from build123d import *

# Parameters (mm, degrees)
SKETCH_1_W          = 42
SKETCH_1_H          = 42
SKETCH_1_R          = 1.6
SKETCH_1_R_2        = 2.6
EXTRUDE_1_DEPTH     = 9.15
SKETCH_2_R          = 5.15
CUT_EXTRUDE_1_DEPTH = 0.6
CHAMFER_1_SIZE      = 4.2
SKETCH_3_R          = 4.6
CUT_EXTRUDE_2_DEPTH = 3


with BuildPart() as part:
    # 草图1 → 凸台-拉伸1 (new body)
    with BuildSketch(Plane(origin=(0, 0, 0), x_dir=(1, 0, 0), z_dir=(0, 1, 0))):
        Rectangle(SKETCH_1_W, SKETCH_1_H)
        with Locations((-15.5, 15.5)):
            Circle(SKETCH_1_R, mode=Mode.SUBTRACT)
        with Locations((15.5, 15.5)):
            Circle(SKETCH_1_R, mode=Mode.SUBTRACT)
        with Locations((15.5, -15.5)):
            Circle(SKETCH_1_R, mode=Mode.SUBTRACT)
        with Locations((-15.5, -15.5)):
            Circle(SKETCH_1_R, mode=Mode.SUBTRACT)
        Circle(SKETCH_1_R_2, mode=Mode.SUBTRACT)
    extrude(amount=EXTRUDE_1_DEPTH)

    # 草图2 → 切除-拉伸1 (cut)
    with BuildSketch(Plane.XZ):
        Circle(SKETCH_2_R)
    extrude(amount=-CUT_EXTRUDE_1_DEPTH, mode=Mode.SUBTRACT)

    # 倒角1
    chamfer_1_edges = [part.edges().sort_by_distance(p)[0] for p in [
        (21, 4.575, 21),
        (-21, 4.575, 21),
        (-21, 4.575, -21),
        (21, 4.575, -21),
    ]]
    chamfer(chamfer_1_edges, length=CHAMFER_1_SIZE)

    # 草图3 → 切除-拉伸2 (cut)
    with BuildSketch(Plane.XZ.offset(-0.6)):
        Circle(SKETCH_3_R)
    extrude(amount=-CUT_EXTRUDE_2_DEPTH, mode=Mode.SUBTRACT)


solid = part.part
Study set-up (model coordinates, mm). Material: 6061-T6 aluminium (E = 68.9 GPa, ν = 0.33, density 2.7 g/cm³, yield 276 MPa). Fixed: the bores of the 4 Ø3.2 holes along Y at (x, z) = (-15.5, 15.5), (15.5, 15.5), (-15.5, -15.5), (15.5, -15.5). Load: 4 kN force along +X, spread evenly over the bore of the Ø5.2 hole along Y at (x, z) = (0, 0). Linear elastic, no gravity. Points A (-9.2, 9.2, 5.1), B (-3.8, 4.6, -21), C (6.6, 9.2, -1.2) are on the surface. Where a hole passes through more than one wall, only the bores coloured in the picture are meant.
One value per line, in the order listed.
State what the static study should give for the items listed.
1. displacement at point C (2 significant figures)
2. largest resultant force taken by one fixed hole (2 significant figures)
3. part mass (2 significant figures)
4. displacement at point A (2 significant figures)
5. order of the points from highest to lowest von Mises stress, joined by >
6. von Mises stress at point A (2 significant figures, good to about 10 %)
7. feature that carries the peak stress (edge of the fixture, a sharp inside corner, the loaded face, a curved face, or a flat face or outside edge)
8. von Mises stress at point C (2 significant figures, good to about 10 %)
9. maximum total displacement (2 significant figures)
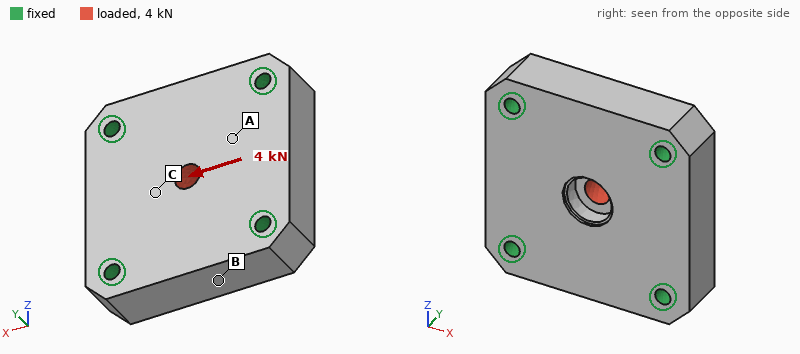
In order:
4.7 µm
1.1 kN
41 g
3.2 µm
C > A > B
17 MPa
the loaded face
25 MPa
7.0 µm
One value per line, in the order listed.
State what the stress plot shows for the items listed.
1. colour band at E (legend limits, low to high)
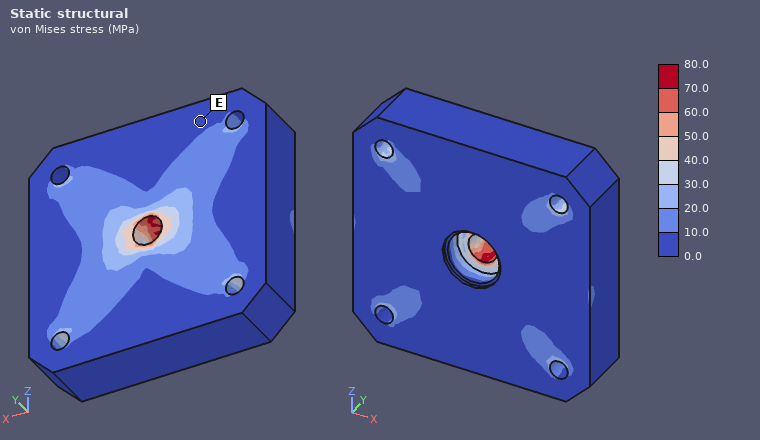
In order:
0.0 to 10.0 MPa
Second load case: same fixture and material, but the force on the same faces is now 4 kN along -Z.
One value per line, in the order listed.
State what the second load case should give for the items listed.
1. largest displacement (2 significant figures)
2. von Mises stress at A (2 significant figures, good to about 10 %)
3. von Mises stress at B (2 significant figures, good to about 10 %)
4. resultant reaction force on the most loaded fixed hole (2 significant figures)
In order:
6.9 µm
14 MPa
8.3 MPa
1.1 kN
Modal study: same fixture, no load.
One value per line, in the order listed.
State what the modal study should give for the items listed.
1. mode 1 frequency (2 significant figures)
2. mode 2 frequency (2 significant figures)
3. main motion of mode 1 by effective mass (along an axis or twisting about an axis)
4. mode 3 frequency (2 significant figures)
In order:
24 kHz
35 kHz
along Y
35 kHz
